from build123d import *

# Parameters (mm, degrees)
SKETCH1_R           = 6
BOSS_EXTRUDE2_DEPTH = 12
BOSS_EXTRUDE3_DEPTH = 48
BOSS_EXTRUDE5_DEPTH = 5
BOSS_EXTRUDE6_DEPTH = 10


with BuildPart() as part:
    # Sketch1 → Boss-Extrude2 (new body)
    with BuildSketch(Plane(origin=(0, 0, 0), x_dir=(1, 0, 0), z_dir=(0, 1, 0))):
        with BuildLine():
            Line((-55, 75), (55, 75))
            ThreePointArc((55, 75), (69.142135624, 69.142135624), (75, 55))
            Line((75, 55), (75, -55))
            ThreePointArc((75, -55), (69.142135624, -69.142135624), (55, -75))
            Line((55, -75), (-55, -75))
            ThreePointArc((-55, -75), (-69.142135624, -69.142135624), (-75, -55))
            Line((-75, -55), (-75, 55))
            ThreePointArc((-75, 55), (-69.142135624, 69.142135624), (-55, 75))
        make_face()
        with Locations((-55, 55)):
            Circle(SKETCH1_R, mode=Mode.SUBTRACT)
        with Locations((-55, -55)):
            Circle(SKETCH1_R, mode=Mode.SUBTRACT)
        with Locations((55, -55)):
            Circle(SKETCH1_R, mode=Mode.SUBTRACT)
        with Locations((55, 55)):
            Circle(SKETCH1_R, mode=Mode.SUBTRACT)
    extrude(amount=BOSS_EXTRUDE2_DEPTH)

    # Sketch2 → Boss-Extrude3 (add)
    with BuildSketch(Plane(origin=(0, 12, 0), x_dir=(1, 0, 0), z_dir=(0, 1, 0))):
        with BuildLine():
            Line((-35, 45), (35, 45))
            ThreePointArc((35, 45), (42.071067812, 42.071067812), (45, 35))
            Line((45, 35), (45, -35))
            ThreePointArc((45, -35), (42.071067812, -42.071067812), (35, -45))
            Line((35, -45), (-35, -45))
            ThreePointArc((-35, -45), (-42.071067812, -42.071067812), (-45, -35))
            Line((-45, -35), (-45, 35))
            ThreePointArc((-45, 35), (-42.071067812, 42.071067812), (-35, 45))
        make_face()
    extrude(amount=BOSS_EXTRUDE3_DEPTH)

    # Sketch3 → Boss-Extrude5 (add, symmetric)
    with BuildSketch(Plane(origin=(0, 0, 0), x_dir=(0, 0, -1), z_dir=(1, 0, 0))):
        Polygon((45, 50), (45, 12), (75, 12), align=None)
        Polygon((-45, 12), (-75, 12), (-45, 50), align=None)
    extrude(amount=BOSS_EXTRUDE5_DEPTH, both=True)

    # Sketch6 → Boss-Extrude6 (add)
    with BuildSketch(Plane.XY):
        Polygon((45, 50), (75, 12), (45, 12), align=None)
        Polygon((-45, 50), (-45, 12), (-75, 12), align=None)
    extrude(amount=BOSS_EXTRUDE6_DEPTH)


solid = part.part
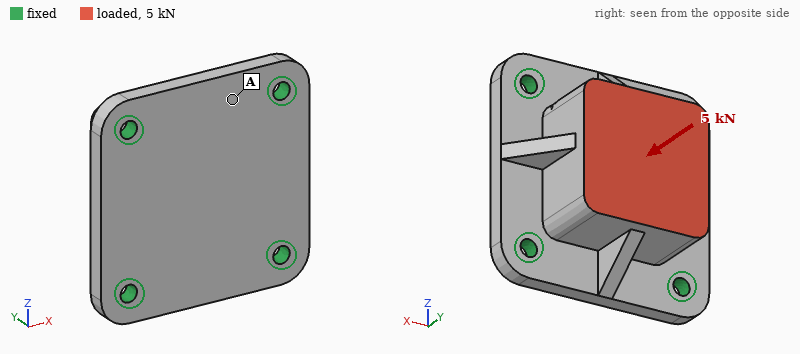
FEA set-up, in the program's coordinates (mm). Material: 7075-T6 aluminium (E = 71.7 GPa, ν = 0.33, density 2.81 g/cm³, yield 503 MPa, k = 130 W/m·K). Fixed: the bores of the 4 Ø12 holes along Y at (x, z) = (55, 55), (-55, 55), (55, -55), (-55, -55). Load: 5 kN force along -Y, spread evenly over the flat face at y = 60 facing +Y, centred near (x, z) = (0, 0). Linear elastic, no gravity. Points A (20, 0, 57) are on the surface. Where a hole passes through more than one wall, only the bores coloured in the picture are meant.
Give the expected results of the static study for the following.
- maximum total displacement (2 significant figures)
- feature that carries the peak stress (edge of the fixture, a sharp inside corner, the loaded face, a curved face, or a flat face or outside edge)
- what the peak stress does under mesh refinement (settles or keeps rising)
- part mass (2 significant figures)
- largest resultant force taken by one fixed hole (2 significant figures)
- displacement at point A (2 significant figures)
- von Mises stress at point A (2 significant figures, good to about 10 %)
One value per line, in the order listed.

7.2 µm
edge of the fixture
keeps rising
1.9 kg
1.3 kN
5.5 µm
2.9 MPa
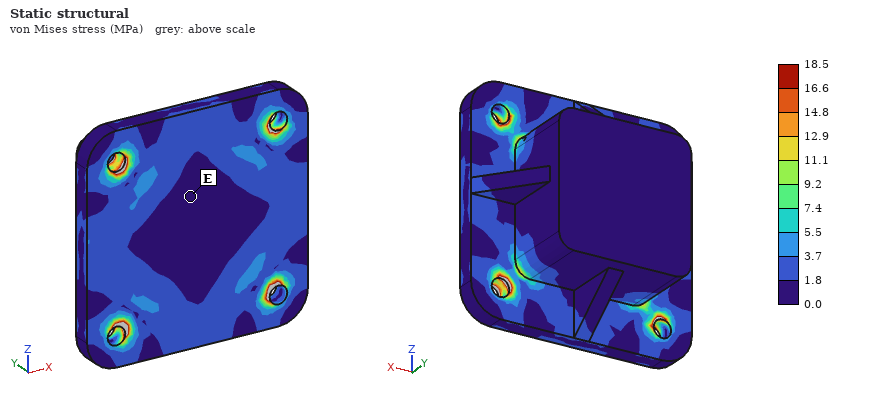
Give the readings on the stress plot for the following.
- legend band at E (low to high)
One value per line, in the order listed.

0.0 to 1.8 MPa
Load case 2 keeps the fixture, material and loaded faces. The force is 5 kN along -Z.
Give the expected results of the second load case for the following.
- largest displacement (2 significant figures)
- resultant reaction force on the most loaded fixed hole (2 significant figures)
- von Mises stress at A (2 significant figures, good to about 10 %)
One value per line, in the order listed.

13 µm
2.0 kN
4.3 MPa
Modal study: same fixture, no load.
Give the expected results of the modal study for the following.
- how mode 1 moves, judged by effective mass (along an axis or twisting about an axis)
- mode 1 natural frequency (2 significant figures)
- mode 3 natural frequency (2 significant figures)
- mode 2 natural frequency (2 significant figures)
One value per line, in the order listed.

along Y
3400 Hz
3900 Hz
3900 Hz
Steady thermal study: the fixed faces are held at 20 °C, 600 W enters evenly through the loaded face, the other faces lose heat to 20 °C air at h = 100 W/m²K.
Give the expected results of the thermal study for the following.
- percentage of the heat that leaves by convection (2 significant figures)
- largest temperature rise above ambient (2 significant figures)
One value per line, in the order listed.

32 %
66 K
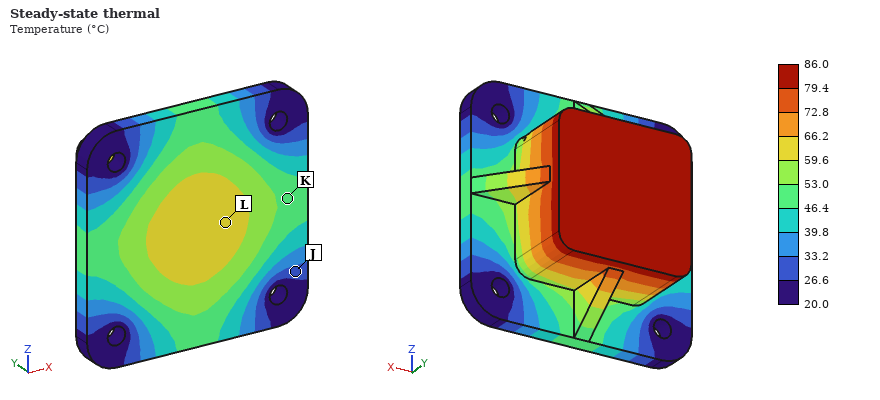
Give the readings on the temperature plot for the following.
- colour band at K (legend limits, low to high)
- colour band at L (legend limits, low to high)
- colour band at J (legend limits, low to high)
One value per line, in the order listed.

46.4 to 53.0 °C
59.6 to 66.2 °C
26.6 to 33.2 °C
